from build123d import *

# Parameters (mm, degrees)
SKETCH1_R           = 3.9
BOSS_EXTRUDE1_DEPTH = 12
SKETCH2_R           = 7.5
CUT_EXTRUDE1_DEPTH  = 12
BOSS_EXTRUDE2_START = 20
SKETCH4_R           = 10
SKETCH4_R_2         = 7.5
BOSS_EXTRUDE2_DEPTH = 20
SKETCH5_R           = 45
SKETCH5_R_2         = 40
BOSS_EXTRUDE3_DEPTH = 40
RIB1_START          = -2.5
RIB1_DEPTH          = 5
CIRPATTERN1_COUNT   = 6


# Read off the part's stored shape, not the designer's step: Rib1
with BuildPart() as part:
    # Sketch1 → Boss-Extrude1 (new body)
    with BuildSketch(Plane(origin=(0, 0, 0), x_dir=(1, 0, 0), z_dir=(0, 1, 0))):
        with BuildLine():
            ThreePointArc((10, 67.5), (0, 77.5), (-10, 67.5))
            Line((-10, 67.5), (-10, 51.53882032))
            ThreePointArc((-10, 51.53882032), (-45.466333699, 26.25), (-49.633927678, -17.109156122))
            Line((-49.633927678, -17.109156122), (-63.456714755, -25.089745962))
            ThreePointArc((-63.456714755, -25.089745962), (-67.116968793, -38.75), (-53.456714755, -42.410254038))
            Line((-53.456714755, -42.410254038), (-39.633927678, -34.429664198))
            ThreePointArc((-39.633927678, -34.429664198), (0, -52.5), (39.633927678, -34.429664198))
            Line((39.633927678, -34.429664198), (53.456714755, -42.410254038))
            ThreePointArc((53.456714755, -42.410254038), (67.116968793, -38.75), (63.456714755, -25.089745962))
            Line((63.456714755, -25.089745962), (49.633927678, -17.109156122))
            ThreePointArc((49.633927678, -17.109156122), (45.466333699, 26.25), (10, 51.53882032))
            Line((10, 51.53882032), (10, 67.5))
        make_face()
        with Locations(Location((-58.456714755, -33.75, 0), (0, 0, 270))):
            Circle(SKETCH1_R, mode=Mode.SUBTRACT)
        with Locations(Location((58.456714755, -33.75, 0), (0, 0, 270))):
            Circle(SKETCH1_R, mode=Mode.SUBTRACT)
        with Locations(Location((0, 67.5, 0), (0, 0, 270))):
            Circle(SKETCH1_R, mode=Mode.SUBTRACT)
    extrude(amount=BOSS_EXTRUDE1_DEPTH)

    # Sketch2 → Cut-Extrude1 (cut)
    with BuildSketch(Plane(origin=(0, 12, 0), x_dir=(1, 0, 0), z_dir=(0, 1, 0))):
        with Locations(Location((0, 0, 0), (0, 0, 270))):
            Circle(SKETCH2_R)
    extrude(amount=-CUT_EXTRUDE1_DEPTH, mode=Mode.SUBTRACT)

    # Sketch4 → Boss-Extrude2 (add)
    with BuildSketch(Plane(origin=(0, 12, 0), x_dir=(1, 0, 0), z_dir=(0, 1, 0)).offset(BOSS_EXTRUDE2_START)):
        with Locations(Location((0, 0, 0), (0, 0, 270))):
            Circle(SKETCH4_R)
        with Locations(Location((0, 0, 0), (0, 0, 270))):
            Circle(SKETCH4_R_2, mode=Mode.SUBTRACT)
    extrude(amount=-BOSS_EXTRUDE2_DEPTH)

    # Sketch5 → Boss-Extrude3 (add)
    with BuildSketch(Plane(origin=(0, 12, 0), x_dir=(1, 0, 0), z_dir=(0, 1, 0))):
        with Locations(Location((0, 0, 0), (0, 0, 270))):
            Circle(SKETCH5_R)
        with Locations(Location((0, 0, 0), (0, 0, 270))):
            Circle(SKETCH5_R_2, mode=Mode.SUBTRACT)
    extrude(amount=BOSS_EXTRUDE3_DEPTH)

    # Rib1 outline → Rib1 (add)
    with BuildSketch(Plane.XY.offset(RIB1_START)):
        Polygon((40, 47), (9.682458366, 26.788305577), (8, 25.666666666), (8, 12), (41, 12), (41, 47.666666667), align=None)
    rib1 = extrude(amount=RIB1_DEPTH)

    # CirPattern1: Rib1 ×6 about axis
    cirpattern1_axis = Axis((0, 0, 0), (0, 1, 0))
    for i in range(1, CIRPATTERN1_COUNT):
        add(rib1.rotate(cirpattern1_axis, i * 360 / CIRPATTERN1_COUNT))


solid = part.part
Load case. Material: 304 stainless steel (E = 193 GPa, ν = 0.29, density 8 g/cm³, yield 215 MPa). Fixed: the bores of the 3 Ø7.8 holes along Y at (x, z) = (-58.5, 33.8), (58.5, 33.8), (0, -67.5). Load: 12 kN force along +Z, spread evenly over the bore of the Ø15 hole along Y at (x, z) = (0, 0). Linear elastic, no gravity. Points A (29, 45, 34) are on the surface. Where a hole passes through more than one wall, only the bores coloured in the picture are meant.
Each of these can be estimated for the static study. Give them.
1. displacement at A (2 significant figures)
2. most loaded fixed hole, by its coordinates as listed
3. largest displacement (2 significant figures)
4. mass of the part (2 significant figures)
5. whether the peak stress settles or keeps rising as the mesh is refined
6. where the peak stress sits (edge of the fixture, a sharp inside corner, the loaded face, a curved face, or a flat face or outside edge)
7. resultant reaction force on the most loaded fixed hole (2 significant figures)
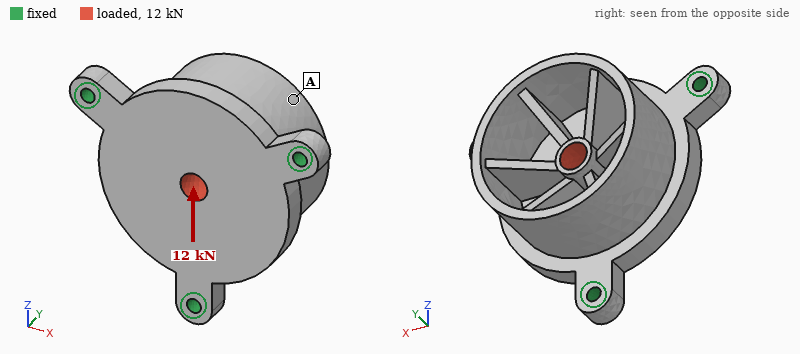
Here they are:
12 µm
(0, -67.5)
18 µm
1.6 kg
keeps rising
edge of the fixture
6.3 kN
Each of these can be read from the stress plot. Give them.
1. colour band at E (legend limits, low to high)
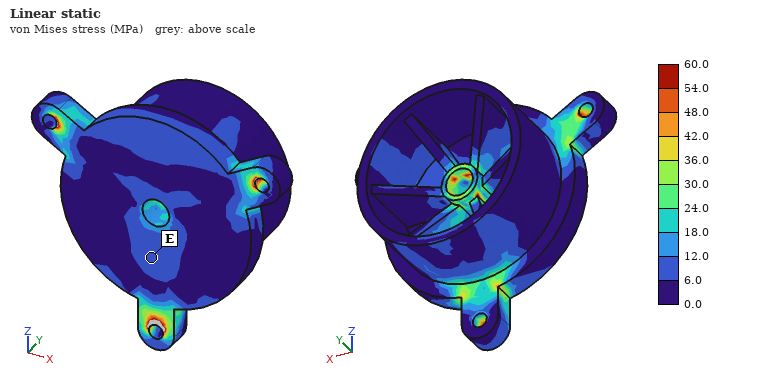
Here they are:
6.0 to 12.0 MPa
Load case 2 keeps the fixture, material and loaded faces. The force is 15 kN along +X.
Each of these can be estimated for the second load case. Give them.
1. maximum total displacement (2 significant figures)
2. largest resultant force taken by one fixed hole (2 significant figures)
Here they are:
20 µm
6.9 kN
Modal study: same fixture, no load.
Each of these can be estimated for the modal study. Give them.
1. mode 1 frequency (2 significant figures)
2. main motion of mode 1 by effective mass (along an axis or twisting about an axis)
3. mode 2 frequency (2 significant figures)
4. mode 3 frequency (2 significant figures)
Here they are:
3200 Hz
along Y
3400 Hz
3400 Hz
